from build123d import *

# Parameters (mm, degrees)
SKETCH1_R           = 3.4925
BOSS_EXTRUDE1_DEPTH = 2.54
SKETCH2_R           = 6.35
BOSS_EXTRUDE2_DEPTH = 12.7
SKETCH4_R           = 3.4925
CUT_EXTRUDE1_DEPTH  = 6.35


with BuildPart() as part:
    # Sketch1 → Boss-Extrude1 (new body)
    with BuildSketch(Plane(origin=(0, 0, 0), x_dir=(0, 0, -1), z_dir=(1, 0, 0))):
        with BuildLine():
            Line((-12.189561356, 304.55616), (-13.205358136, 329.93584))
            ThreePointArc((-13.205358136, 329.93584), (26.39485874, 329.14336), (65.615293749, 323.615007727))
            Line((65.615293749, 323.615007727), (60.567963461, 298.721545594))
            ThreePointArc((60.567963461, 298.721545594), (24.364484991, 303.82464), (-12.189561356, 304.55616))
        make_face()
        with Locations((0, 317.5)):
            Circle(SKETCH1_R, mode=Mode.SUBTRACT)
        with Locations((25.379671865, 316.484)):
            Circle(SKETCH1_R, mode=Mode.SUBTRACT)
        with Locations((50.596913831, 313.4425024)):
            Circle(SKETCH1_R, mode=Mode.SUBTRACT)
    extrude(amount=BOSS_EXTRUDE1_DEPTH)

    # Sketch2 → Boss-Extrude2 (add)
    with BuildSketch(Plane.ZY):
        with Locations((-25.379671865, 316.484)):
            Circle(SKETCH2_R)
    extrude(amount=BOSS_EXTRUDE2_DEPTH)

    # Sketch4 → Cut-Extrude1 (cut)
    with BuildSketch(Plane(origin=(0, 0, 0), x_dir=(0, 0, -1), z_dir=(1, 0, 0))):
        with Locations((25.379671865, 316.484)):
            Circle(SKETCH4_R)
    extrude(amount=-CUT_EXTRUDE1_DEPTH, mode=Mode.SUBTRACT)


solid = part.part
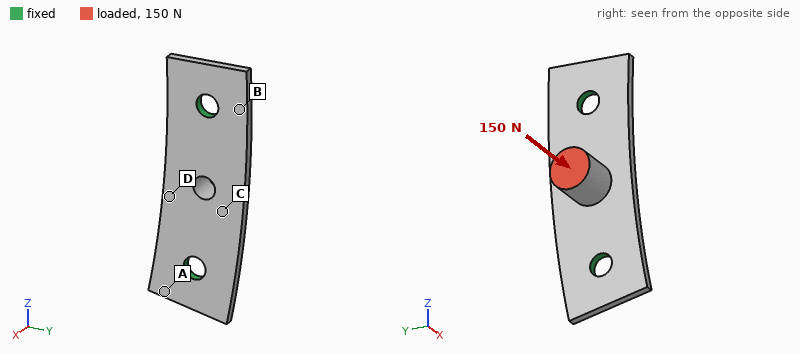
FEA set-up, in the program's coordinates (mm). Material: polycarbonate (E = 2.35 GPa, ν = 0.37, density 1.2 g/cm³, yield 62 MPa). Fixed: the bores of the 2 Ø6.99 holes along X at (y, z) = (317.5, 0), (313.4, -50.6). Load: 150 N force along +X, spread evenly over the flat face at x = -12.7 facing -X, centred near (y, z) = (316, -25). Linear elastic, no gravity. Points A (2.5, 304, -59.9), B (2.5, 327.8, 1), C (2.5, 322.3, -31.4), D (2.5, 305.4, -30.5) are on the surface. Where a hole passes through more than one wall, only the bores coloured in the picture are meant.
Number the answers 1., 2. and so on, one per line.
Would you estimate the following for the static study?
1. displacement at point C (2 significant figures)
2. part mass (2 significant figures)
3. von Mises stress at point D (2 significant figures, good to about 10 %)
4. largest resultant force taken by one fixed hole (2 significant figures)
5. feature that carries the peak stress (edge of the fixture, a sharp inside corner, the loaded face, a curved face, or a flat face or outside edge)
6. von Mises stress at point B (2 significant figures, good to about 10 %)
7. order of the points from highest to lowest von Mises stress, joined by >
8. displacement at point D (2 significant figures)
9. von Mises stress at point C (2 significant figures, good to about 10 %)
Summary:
1. 0.66 mm
2. 7.2 g
3. 12 MPa
4. 81 N
5. a flat face or outside edge
6. 6.6 MPa
7. C > D > B > A
8. 0.56 mm
9. 15 MPa
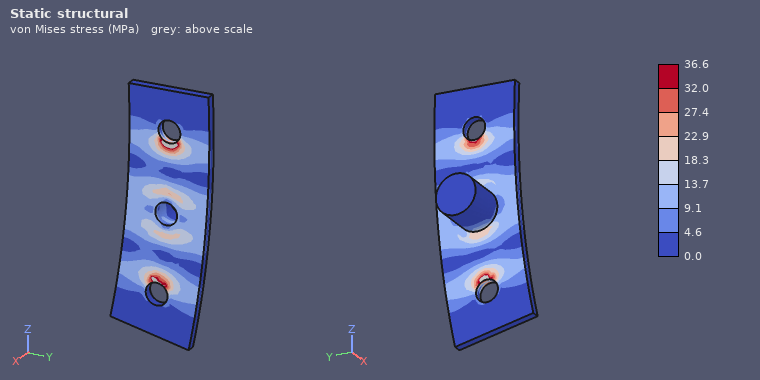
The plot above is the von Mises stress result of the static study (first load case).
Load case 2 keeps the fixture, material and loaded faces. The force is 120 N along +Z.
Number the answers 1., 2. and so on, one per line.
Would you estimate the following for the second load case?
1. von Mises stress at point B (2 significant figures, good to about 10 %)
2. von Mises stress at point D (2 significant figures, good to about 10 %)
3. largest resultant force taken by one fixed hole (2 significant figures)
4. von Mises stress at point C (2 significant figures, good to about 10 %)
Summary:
1. 2.2 MPa
2. 9.4 MPa
3. 79 N
4. 14 MPa
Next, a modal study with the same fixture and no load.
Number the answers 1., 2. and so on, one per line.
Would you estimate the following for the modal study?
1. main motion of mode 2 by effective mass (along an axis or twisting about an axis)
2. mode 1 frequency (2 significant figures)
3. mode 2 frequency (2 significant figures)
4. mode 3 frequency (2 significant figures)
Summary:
1. along X
2. 1200 Hz
3. 1300 Hz
4. 2500 Hz
